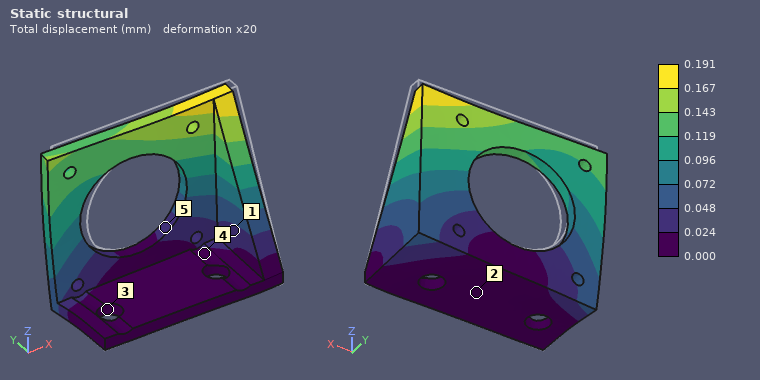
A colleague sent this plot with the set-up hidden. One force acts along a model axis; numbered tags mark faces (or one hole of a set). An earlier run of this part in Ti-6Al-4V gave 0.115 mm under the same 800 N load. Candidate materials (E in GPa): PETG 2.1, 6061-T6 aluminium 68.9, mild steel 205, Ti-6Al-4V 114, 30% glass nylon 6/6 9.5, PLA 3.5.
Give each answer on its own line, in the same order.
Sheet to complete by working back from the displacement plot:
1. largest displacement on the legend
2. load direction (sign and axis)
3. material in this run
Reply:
0.191 mm
-X
6061-T6 aluminium
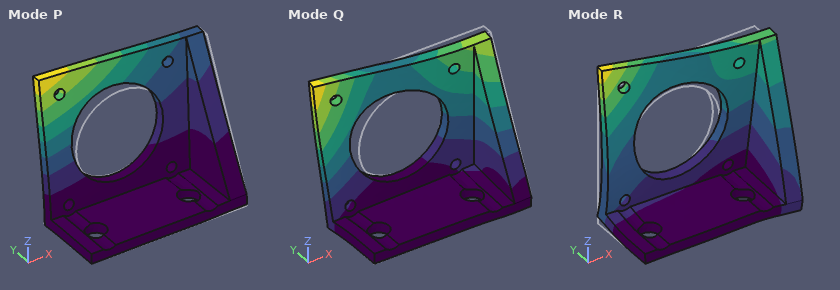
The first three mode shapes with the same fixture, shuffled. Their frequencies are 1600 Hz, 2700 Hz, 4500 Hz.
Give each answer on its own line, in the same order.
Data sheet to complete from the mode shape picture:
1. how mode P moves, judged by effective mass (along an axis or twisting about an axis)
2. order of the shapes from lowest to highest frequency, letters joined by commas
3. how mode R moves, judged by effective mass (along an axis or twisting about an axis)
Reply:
along Y
P, Q, R
along X
